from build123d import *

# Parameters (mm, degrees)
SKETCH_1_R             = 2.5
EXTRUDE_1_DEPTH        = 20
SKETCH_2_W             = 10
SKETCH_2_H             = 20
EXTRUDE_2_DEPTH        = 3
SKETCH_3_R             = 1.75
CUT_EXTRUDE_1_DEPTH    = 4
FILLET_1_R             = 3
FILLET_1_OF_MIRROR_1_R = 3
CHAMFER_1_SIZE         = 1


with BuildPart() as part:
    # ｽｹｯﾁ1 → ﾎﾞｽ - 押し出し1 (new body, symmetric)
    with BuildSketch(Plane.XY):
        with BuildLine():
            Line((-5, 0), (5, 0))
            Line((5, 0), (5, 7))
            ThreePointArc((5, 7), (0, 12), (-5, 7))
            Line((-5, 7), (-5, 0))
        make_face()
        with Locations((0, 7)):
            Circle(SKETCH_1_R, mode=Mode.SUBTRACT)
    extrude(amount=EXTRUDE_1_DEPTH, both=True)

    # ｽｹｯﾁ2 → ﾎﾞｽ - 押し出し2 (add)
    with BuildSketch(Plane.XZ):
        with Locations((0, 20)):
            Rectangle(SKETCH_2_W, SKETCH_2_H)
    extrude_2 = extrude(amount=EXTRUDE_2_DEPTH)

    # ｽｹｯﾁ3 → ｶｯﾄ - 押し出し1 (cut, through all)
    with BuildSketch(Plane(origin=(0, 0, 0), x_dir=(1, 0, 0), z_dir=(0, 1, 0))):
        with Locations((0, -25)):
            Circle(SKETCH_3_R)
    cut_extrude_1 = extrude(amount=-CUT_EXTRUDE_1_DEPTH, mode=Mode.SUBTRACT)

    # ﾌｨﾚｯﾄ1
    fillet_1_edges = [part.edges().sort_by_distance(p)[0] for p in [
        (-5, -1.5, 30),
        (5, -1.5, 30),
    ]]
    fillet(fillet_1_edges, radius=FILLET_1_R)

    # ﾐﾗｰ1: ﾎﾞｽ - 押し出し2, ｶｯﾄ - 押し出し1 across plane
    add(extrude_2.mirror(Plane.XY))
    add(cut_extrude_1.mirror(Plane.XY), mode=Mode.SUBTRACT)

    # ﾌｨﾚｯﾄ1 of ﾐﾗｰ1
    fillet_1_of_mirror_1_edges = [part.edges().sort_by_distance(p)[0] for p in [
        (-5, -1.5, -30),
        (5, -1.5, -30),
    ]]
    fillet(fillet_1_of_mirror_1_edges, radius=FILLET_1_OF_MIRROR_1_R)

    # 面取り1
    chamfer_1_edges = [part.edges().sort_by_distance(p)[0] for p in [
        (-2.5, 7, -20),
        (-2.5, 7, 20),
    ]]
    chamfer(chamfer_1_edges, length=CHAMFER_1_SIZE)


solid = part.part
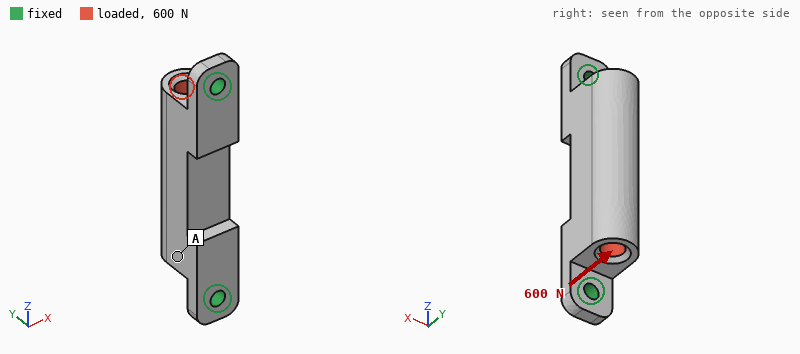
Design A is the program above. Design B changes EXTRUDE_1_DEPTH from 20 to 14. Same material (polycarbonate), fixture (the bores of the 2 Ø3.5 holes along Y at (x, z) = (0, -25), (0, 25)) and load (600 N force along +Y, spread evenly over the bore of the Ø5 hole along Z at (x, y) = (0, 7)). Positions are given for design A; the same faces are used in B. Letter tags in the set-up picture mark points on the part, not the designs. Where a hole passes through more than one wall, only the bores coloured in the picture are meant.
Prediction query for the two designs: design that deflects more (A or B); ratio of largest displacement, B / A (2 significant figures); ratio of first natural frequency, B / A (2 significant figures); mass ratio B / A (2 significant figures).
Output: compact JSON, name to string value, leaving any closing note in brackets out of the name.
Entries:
{"design that deflects more": "B", "ratio of largest displacement, B / A": "3.4", "ratio of first natural frequency, B / A": "0.76", "mass ratio B / A": "0.77"}
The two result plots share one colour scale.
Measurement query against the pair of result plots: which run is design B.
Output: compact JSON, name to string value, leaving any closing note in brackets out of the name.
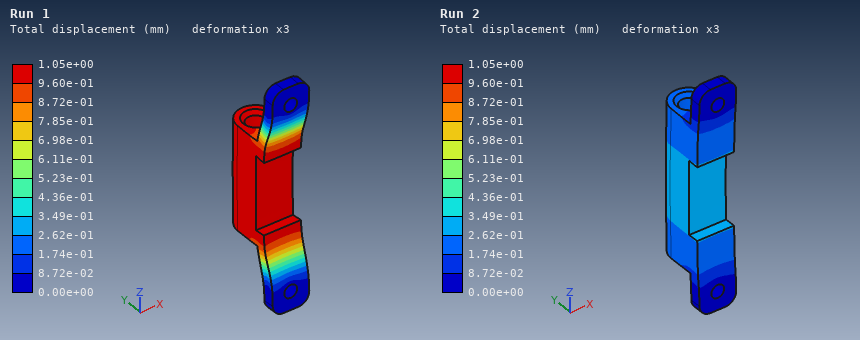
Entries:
{"which run is design B": "Run 1"}
